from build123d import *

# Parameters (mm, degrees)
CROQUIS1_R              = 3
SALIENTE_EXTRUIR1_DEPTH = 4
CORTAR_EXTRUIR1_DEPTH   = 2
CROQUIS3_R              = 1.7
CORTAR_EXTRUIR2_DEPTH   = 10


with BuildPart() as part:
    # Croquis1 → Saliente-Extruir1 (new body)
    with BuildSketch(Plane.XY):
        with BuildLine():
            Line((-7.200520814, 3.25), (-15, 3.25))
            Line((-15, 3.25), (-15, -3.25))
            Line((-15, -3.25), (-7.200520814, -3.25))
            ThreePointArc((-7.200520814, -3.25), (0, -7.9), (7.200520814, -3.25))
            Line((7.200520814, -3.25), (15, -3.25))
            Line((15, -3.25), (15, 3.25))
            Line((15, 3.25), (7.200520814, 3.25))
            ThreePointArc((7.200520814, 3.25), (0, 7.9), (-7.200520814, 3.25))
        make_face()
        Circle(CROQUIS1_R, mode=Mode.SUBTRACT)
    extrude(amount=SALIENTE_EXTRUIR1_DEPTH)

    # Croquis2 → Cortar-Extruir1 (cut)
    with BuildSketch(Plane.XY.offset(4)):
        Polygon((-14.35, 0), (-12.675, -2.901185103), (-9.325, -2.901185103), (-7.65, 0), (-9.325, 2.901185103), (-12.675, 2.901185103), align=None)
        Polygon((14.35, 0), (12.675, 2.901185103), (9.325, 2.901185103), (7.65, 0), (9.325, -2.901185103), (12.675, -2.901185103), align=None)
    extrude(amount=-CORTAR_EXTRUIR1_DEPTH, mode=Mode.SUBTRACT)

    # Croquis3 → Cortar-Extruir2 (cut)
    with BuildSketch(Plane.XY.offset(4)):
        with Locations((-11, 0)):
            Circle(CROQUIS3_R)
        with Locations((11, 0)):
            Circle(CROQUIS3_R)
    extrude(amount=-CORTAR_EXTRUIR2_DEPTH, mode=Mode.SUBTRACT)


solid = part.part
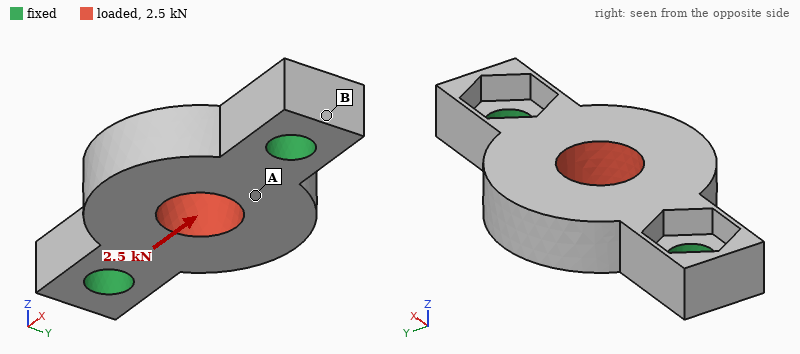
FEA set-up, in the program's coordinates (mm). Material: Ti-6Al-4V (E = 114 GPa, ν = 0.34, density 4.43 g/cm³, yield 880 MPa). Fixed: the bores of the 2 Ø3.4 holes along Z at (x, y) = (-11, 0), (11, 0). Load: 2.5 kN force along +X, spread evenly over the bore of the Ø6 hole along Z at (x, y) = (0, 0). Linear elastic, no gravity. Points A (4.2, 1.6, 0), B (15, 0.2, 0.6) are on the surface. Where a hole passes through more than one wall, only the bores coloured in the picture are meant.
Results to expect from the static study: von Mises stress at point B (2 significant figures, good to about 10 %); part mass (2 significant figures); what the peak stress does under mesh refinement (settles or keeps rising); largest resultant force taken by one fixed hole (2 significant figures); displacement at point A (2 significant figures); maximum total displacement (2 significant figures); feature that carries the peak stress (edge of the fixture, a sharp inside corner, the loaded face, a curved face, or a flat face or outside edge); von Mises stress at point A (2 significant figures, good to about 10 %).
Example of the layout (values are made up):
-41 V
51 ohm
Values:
19 MPa
4.0 g
keeps rising
1.3 kN
3.6 µm
5.5 µm
edge of the fixture
66 MPa
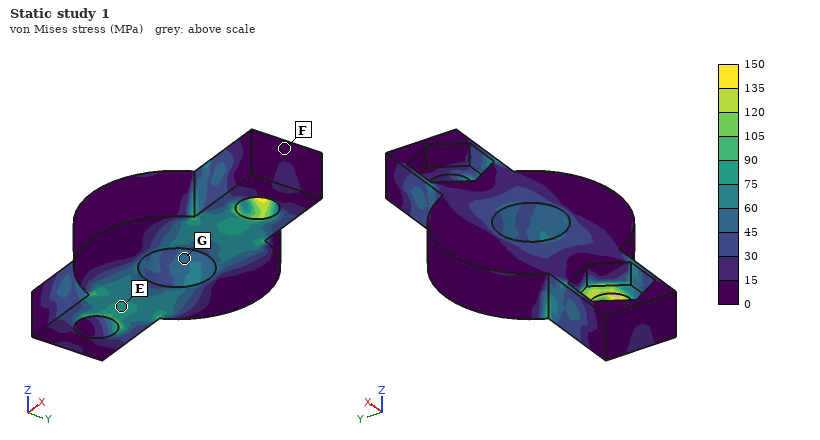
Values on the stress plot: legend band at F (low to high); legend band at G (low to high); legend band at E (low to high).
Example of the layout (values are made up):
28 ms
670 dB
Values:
0 to 15 MPa
45 to 60 MPa
75 to 90 MPa
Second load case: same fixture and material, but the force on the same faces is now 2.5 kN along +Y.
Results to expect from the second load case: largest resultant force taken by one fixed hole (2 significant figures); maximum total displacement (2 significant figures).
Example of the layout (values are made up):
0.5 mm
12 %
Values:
1.3 kN
28 µm
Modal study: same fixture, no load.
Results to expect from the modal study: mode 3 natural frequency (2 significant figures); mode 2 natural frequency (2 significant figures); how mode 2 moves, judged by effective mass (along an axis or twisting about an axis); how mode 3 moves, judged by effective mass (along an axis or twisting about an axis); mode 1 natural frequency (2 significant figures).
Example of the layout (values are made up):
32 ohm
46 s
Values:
45 kHz
24 kHz
along Z
along Y
18 kHz
